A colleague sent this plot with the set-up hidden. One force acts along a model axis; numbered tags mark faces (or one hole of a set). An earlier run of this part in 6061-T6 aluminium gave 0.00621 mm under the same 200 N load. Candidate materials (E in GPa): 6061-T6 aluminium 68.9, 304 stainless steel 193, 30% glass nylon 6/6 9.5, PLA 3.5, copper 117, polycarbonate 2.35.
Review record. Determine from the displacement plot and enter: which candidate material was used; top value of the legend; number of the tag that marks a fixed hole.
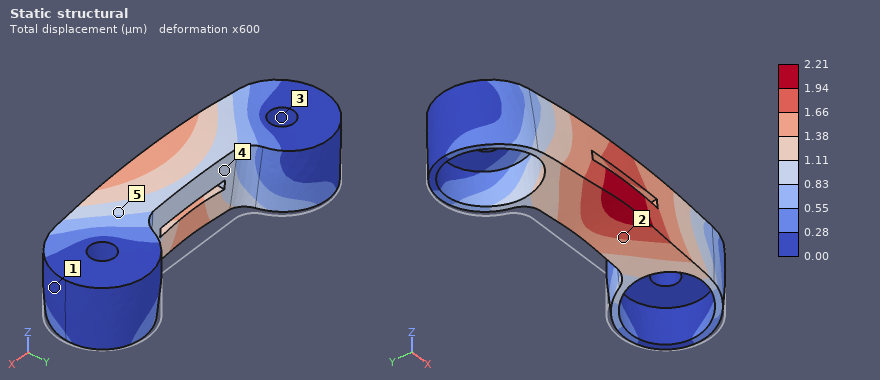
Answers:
304 stainless steel
2.21 µm
3
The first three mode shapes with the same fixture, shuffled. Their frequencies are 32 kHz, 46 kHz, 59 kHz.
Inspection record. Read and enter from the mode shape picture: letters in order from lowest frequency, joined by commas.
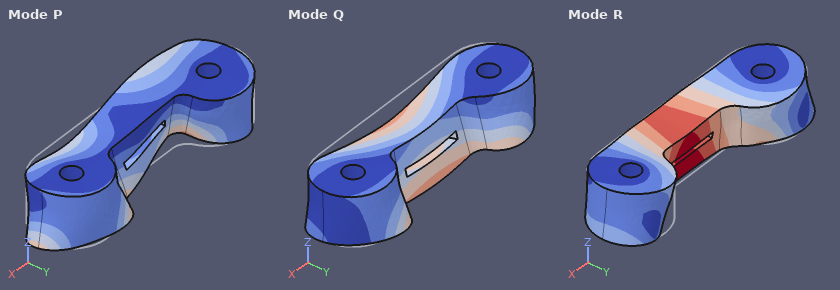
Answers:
Q, R, P
